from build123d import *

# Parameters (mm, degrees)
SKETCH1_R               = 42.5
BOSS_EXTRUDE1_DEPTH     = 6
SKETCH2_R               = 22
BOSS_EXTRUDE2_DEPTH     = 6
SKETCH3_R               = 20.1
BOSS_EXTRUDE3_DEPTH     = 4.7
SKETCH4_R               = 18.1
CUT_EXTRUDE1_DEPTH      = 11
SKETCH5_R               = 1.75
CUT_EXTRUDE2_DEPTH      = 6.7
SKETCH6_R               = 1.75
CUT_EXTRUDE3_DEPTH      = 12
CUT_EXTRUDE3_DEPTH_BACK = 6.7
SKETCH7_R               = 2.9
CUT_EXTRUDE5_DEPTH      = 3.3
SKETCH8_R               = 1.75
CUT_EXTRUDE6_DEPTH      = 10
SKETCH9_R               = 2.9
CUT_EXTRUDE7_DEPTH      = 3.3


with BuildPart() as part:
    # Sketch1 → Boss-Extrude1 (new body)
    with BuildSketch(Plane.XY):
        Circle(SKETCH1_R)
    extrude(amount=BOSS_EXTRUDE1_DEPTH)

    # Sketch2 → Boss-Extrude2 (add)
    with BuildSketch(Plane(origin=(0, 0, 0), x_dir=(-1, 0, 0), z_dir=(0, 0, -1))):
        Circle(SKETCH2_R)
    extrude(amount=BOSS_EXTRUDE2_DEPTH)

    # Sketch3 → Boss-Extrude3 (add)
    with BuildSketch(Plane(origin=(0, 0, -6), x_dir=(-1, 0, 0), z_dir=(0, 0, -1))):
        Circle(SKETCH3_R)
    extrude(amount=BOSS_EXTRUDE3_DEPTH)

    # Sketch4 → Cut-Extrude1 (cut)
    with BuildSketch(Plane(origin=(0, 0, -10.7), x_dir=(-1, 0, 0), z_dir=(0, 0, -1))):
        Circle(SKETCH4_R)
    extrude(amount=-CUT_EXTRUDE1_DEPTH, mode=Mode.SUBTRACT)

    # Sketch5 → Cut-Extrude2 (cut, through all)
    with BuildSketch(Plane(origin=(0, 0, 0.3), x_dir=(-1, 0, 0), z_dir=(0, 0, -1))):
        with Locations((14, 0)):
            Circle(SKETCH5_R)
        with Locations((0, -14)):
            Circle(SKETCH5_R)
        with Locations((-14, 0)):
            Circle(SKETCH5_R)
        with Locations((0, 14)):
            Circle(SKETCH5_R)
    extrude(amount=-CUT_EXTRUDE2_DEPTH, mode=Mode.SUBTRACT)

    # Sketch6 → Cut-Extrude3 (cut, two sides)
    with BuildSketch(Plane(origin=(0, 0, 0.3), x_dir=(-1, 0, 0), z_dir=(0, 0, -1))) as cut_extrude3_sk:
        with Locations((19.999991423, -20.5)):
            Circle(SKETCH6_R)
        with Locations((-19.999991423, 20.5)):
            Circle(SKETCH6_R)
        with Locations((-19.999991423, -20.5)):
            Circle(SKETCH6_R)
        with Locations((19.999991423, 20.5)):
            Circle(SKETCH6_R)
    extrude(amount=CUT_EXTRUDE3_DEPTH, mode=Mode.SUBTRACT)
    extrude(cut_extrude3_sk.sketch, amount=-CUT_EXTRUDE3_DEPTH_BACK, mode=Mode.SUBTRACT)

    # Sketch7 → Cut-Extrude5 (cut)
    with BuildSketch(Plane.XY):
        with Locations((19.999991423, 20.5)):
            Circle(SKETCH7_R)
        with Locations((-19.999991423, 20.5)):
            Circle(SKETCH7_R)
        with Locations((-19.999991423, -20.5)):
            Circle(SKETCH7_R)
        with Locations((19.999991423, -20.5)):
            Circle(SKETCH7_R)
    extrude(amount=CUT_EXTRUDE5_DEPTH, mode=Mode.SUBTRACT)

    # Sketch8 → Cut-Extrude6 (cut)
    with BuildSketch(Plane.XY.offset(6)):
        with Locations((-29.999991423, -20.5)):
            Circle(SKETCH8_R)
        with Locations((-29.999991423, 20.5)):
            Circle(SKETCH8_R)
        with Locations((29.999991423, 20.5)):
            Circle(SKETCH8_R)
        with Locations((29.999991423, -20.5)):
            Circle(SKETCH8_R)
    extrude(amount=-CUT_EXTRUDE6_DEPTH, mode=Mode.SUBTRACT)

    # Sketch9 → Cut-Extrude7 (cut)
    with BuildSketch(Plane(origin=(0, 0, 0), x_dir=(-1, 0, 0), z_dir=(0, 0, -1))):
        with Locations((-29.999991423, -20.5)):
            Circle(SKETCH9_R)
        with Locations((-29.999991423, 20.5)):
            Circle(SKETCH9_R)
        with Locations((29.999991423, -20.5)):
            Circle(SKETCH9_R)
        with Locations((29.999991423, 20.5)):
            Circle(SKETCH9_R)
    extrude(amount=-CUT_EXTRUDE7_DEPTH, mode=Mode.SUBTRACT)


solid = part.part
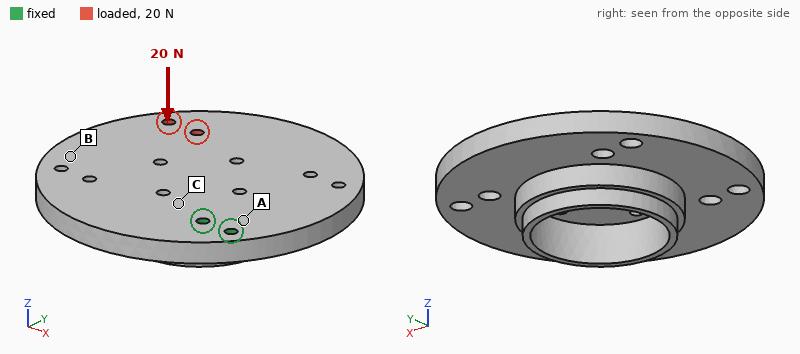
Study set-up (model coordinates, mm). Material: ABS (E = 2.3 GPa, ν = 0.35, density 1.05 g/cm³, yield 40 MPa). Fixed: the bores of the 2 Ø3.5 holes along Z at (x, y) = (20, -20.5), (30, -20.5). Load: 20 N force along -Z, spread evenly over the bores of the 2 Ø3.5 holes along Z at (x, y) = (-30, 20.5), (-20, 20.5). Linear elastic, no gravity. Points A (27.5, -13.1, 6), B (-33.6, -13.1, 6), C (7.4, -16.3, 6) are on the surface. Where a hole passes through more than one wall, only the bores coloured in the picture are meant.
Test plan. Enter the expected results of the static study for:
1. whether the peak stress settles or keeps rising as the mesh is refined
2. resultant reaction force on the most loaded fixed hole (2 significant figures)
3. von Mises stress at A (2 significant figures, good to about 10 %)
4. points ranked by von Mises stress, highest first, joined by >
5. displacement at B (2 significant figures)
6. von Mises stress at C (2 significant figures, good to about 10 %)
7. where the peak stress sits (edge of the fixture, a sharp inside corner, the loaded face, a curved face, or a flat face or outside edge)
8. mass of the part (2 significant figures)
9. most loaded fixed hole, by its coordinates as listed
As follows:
keeps rising
88 N
3.4 MPa
A > C > B
0.57 mm
2.1 MPa
edge of the fixture
39 g
(20, -20.5)
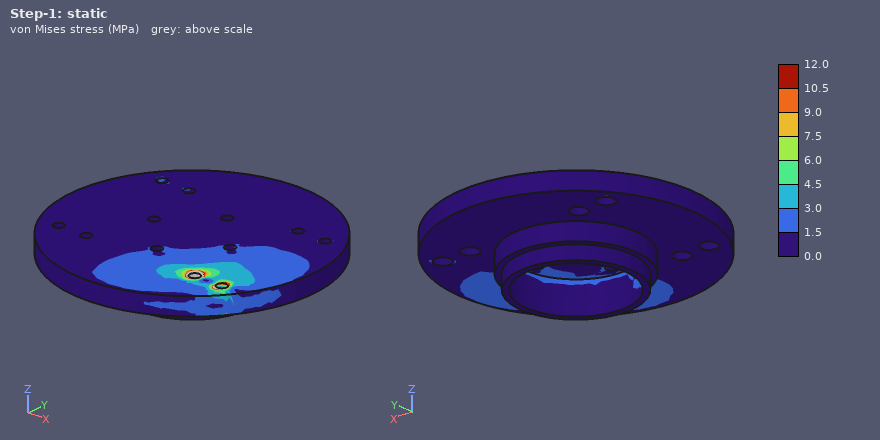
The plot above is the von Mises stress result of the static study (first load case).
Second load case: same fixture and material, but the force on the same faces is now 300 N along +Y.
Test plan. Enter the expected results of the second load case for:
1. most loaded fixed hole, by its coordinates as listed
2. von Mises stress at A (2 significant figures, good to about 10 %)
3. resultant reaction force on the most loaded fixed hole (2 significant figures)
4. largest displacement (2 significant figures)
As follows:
(20, -20.5)
15 MPa
1.4 kN
1.4 mm
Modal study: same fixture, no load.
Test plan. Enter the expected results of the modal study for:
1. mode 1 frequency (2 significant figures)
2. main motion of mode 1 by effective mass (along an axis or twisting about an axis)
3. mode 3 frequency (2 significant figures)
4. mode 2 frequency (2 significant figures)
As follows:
200 Hz
along Z
530 Hz
390 Hz
